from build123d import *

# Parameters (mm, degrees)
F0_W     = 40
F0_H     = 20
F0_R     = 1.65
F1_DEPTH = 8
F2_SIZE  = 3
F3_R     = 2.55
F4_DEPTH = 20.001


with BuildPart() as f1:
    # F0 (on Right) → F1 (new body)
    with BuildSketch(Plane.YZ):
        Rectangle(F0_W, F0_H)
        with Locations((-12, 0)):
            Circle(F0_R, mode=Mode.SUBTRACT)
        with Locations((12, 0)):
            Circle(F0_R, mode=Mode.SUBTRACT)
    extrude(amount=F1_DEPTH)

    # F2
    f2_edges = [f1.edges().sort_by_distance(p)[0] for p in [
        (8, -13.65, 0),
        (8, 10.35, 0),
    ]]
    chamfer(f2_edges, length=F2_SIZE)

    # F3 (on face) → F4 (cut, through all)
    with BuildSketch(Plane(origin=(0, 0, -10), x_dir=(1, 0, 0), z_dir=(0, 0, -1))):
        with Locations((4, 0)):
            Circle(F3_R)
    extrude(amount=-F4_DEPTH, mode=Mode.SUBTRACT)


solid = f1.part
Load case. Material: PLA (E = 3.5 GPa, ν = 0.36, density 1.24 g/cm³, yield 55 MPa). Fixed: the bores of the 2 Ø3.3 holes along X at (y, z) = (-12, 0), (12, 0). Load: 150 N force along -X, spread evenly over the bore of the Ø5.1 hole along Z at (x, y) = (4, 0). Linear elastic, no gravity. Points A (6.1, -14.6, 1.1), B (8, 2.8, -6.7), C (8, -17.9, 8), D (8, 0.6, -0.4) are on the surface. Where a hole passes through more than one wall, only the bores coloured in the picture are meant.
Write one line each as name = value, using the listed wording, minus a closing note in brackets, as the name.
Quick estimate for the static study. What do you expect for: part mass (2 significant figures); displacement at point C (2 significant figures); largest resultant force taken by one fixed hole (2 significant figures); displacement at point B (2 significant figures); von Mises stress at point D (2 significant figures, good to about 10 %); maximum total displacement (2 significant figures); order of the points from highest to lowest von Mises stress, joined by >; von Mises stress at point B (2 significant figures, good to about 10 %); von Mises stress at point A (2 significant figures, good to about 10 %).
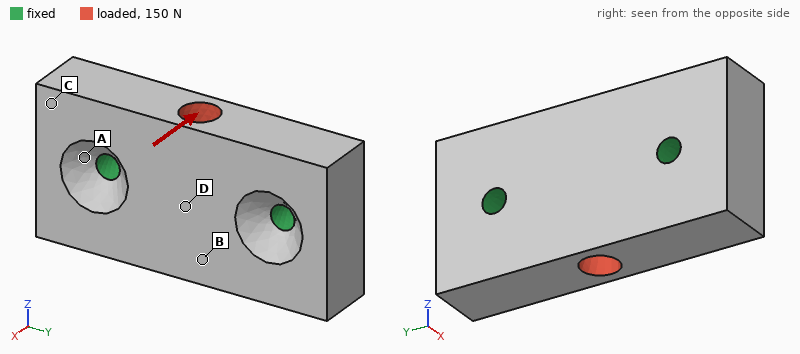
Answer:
part mass = 7.1 g
displacement at point C = 4.1 µm
largest resultant force taken by one fixed hole = 79 N
displacement at point B = 13 µm
von Mises stress at point D = 3.2 MPa
maximum total displacement = 17 µm
order of the points from highest to lowest von Mises stress, joined by > = D > B > A > C
von Mises stress at point B = 2.4 MPa
von Mises stress at point A = 1.3 MPa
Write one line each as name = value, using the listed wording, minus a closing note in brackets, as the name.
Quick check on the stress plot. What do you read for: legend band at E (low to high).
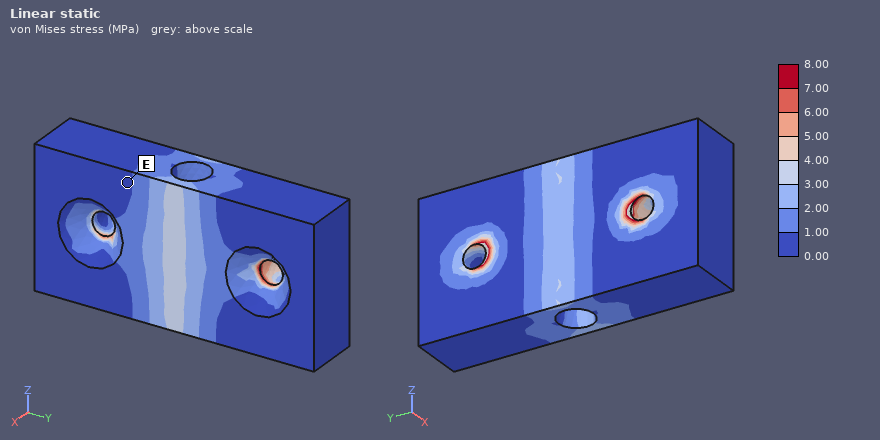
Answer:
legend band at E = 0.00 to 1.00 MPa
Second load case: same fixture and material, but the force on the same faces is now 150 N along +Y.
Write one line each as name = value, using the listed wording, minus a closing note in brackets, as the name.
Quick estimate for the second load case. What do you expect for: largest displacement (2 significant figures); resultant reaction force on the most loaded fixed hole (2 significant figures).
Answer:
largest displacement = 3.3 µm
resultant reaction force on the most loaded fixed hole = 75 N
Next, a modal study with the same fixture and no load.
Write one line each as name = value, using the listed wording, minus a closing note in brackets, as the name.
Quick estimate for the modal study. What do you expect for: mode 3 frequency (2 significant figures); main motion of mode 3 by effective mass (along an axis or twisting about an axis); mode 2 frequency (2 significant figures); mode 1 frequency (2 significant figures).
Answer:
mode 3 frequency = 11 kHz
main motion of mode 3 by effective mass = along X
mode 2 frequency = 10 kHz
mode 1 frequency = 7100 Hz
